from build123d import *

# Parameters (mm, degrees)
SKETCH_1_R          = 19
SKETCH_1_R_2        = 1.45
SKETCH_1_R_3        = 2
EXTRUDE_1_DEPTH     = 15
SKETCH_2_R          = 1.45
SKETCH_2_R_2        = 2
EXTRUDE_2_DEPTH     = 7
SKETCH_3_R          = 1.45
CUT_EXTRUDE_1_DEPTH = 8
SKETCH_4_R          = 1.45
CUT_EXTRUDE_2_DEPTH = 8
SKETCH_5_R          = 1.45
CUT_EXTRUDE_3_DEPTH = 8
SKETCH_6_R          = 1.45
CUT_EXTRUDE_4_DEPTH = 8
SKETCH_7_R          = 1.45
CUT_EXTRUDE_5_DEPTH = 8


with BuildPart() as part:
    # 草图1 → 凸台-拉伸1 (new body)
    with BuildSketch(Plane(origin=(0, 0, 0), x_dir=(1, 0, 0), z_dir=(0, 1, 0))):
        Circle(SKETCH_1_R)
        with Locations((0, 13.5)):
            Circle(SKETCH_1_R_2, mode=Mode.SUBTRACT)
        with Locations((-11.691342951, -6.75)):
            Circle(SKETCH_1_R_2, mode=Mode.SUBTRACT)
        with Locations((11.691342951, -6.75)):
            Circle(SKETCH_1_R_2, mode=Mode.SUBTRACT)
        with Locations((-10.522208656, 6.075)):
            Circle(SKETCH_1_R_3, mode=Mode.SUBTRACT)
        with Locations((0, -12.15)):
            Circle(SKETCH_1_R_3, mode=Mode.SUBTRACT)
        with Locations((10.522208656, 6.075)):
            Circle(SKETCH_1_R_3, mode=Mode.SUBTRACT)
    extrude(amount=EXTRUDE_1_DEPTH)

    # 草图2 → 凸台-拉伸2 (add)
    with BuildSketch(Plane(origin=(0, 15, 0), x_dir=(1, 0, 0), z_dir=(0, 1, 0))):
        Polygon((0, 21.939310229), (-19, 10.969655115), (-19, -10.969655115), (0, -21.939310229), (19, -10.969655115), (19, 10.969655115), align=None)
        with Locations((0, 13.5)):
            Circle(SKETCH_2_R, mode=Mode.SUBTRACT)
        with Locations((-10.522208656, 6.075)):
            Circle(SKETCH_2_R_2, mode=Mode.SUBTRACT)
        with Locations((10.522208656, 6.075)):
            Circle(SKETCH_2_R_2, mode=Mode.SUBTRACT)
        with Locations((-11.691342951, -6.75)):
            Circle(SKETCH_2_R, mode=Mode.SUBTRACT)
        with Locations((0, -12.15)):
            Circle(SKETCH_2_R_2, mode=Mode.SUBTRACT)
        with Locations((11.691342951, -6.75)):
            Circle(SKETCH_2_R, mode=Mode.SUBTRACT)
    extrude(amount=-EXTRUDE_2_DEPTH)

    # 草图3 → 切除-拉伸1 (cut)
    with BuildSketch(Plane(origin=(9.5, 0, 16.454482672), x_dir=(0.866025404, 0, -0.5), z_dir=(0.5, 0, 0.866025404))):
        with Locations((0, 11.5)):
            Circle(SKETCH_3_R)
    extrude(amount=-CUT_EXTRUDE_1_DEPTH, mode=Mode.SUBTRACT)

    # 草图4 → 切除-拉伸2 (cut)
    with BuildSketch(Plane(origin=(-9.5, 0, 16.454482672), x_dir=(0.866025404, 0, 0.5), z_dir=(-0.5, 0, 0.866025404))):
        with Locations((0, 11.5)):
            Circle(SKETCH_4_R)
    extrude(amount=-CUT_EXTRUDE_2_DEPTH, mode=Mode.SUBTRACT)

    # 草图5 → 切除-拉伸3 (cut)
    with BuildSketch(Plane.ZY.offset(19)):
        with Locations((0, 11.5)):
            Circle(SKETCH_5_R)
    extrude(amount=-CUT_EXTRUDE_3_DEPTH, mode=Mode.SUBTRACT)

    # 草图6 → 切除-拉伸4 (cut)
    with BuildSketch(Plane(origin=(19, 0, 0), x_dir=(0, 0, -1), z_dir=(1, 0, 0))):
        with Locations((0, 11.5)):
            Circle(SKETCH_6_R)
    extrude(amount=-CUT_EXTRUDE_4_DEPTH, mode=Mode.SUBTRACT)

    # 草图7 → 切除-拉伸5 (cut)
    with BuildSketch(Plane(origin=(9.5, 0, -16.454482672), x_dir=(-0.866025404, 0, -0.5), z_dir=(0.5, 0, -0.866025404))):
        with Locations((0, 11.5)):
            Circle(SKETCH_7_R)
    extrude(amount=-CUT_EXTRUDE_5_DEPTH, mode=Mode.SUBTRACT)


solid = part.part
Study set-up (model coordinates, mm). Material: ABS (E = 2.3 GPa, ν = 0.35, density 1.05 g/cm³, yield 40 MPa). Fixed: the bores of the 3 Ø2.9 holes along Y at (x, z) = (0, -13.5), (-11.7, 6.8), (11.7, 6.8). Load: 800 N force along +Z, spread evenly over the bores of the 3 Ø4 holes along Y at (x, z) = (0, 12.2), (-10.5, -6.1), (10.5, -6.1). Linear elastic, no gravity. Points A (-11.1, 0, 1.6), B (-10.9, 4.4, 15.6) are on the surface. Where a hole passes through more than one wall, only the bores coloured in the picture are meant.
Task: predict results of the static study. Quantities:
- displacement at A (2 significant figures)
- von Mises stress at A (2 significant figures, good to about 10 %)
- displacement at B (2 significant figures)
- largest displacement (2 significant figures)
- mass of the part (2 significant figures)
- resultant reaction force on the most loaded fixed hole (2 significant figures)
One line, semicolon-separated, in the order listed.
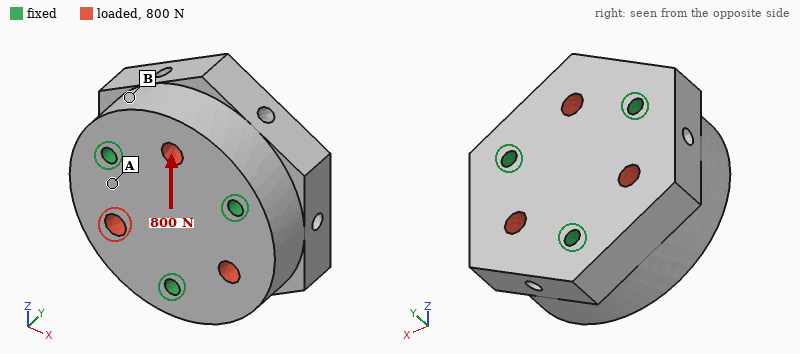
3.7 µm; 1.7 MPa; 2.9 µm; 11 µm; 18 g; 280 N
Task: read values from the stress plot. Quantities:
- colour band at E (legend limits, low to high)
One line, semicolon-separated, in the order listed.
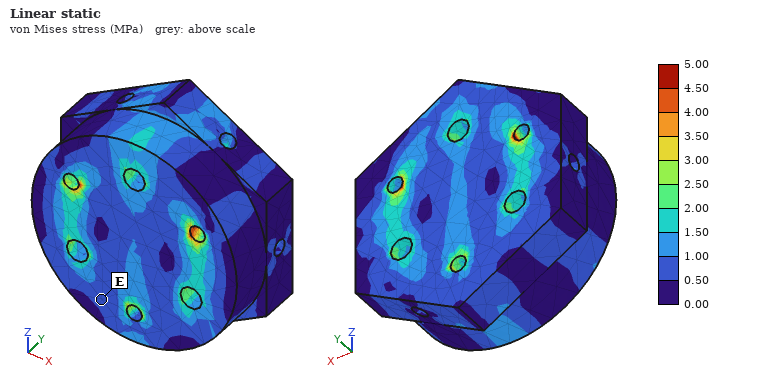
0.50 to 1.00 MPa
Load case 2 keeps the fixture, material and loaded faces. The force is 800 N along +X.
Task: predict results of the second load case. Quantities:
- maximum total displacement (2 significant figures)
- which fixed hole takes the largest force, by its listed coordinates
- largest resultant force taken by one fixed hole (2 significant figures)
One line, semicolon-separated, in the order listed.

11 µm; (0, -13.5); 300 N
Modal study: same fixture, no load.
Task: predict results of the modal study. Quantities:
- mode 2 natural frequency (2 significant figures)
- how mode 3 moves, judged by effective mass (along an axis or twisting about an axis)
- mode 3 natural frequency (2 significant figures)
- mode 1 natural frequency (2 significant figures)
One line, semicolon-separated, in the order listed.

11 kHz; along Y; 12 kHz; 11 kHz
